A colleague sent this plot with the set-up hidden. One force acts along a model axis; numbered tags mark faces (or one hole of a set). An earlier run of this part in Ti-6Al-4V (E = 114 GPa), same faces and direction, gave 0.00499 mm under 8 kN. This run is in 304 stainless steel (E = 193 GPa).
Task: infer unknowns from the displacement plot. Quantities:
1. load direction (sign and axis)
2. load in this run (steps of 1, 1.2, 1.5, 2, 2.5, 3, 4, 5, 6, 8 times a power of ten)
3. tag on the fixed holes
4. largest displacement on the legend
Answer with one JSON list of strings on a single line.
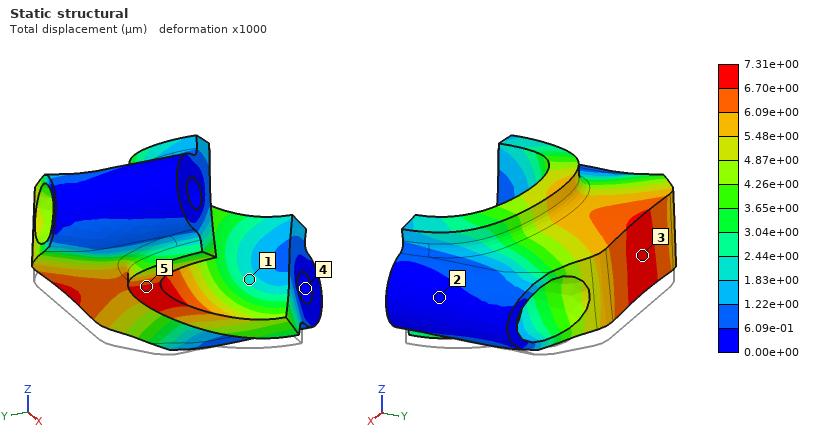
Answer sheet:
["+Z", "20 kN", "4", "7.31e+00 µm"]
